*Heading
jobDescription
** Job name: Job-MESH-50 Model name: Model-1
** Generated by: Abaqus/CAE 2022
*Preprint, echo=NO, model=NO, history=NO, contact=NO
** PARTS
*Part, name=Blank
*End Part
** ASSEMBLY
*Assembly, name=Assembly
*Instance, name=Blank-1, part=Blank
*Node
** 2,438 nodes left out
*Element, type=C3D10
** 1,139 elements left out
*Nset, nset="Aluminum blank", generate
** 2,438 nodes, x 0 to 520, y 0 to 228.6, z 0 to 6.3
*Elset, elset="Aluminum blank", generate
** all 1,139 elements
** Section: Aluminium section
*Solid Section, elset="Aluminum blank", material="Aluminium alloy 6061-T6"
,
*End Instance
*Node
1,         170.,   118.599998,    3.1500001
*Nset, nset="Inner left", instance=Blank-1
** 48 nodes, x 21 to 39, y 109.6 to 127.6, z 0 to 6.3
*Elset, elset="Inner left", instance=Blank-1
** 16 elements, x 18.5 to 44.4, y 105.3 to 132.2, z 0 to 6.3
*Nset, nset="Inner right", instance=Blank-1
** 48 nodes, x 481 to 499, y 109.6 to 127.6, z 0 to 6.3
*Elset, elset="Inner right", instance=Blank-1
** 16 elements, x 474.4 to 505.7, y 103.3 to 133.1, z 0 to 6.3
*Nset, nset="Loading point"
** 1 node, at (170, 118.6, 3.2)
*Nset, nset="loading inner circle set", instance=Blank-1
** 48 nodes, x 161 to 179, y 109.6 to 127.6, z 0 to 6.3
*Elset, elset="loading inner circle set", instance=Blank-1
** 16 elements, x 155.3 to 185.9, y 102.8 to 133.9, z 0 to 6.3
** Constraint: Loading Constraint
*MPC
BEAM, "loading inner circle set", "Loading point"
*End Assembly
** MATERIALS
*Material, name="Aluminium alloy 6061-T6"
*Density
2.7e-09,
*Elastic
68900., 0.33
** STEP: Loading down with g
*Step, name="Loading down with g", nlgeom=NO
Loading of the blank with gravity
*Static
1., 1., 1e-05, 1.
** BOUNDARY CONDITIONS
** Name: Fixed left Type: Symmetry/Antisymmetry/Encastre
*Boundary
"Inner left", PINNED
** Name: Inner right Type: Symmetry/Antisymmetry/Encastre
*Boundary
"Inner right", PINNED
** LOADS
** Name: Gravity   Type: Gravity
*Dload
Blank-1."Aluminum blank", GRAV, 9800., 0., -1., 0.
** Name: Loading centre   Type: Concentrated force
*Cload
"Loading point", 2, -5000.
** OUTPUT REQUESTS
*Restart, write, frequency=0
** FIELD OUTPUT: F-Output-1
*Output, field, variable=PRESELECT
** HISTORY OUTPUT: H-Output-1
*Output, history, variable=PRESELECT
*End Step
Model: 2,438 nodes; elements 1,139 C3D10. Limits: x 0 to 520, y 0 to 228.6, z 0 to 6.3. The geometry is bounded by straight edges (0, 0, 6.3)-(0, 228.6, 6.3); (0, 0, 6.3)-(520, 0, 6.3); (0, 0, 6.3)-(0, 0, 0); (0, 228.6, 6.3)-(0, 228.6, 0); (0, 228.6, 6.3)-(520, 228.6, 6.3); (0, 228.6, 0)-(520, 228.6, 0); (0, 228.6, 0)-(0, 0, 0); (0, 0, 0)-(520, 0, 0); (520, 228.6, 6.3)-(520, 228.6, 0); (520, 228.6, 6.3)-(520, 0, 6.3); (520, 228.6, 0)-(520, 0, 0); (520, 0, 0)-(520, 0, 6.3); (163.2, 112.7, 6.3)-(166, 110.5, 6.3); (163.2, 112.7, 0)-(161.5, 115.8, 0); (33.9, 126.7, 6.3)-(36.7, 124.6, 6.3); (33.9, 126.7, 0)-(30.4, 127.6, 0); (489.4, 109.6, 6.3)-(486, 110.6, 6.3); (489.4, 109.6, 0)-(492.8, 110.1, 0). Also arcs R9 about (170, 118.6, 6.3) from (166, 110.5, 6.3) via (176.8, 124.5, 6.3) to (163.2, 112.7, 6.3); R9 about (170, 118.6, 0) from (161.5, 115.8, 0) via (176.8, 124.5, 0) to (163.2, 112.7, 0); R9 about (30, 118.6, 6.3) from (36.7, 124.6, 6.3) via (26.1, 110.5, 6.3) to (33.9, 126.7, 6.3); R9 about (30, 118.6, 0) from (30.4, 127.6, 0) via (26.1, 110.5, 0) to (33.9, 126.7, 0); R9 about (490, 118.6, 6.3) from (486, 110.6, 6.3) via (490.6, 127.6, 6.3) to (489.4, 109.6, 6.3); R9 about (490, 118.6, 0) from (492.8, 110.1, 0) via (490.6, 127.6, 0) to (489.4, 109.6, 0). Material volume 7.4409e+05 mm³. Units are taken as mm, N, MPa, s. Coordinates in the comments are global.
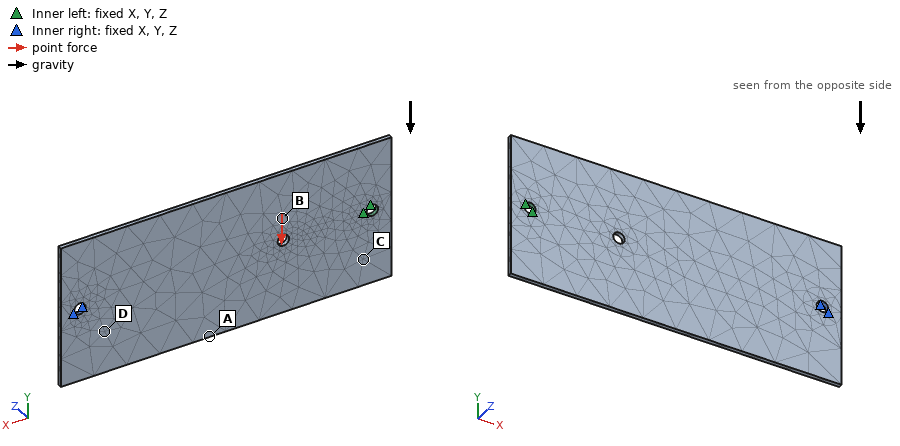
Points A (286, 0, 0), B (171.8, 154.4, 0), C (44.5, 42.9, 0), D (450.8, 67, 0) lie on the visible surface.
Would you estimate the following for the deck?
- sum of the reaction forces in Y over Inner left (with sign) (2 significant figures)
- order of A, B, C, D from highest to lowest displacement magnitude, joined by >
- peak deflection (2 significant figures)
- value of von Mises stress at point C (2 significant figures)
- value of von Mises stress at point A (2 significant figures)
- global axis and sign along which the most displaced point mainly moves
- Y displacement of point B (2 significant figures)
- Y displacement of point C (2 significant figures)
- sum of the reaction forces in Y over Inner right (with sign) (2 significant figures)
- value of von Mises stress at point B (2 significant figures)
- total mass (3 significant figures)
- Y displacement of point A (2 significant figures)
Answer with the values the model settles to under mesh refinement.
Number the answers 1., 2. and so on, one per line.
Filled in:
1. 3500 N
2. B > A > C > D
3. 0.037 mm
4. 2.5 MPa
5. 5.6 MPa
6. -Y
7. -0.033 mm
8. -0.0066 mm
9. 1500 N
10. 6.8 MPa
11. 2.01 kg
12. -0.027 mm
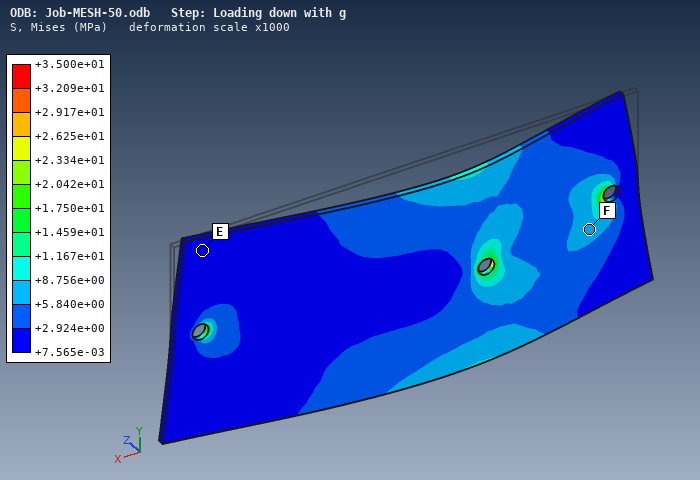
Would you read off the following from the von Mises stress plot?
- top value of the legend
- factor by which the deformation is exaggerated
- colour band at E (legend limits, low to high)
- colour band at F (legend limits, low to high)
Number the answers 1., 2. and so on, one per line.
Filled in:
1. +3.500e+01 MPa
2. 1000
3. +7.565e-03 to +2.924e+00 MPa
4. +5.840e+00 to +8.756e+00 MPa
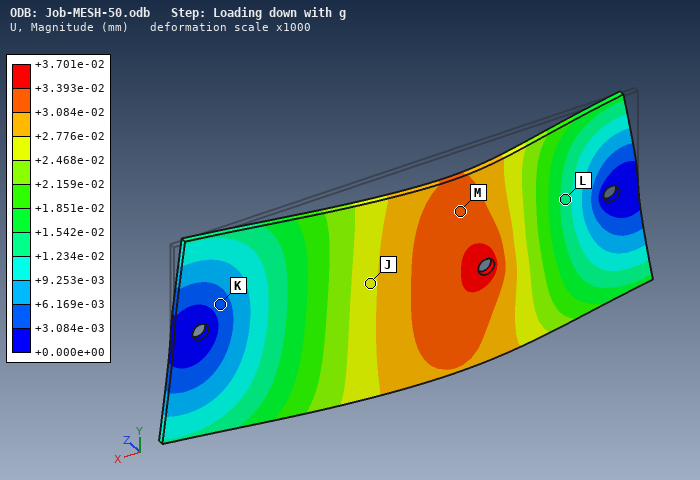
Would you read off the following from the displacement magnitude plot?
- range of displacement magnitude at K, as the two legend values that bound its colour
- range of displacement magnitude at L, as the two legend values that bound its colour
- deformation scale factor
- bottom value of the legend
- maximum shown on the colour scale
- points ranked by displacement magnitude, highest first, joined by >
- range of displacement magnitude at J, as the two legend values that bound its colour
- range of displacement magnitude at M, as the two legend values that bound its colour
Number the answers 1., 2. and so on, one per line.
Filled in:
1. +3.084e-03 to +6.169e-03 mm
2. +1.234e-02 to +1.542e-02 mm
3. 1000
4. +0.000e+00 mm
5. +3.701e-02 mm
6. M > J > L > K
7. +2.468e-02 to +2.776e-02 mm
8. +3.084e-02 to +3.393e-02 mm
